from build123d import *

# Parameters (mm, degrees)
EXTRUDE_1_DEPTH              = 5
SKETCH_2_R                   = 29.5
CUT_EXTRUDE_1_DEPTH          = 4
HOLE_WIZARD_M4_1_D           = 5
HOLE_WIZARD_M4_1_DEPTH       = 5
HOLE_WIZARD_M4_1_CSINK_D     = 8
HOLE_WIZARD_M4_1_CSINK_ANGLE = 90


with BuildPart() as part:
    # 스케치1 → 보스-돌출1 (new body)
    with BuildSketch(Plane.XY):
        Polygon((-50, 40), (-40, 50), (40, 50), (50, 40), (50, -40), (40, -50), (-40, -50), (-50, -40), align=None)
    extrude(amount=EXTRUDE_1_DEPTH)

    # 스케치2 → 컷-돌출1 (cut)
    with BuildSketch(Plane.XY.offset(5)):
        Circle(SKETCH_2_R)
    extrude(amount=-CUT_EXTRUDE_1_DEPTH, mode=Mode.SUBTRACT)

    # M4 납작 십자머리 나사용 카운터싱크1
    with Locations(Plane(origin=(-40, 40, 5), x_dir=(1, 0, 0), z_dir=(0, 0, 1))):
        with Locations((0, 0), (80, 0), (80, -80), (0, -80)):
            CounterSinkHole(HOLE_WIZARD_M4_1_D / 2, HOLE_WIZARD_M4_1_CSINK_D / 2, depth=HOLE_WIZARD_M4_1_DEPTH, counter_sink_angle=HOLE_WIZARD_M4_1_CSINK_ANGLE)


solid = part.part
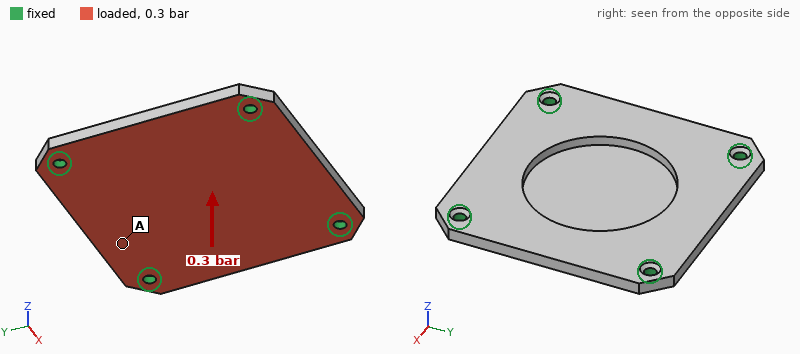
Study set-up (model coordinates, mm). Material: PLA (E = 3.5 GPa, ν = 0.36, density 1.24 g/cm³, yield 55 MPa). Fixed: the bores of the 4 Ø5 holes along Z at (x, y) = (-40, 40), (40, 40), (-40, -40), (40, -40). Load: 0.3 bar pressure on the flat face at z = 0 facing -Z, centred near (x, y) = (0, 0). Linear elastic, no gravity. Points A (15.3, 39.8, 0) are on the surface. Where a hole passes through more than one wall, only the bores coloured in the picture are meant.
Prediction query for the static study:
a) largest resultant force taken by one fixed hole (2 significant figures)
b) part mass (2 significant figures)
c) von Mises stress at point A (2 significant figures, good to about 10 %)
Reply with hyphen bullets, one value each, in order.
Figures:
- 77 N
- 47 g
- 1.8 MPa
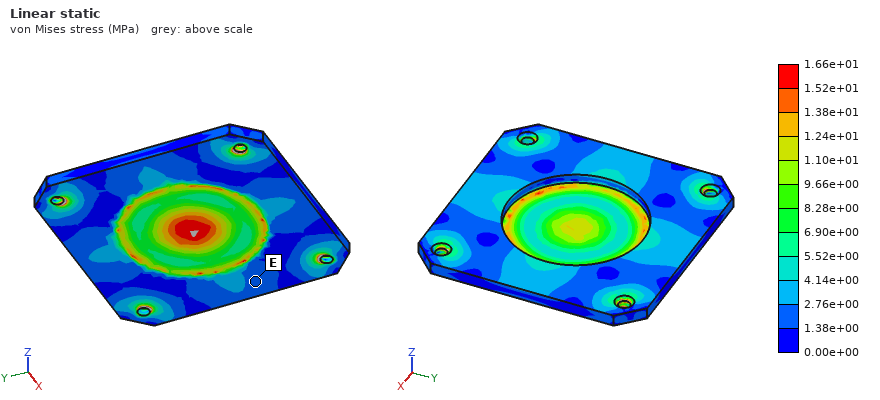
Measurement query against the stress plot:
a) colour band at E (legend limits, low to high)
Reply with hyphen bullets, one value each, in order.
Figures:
- 1.38e+00 to 2.76e+00 MPa
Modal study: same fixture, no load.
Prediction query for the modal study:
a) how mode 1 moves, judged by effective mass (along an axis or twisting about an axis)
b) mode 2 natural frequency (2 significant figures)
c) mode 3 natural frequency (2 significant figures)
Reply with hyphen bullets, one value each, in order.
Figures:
- along Z
- 1300 Hz
- 1300 Hz
